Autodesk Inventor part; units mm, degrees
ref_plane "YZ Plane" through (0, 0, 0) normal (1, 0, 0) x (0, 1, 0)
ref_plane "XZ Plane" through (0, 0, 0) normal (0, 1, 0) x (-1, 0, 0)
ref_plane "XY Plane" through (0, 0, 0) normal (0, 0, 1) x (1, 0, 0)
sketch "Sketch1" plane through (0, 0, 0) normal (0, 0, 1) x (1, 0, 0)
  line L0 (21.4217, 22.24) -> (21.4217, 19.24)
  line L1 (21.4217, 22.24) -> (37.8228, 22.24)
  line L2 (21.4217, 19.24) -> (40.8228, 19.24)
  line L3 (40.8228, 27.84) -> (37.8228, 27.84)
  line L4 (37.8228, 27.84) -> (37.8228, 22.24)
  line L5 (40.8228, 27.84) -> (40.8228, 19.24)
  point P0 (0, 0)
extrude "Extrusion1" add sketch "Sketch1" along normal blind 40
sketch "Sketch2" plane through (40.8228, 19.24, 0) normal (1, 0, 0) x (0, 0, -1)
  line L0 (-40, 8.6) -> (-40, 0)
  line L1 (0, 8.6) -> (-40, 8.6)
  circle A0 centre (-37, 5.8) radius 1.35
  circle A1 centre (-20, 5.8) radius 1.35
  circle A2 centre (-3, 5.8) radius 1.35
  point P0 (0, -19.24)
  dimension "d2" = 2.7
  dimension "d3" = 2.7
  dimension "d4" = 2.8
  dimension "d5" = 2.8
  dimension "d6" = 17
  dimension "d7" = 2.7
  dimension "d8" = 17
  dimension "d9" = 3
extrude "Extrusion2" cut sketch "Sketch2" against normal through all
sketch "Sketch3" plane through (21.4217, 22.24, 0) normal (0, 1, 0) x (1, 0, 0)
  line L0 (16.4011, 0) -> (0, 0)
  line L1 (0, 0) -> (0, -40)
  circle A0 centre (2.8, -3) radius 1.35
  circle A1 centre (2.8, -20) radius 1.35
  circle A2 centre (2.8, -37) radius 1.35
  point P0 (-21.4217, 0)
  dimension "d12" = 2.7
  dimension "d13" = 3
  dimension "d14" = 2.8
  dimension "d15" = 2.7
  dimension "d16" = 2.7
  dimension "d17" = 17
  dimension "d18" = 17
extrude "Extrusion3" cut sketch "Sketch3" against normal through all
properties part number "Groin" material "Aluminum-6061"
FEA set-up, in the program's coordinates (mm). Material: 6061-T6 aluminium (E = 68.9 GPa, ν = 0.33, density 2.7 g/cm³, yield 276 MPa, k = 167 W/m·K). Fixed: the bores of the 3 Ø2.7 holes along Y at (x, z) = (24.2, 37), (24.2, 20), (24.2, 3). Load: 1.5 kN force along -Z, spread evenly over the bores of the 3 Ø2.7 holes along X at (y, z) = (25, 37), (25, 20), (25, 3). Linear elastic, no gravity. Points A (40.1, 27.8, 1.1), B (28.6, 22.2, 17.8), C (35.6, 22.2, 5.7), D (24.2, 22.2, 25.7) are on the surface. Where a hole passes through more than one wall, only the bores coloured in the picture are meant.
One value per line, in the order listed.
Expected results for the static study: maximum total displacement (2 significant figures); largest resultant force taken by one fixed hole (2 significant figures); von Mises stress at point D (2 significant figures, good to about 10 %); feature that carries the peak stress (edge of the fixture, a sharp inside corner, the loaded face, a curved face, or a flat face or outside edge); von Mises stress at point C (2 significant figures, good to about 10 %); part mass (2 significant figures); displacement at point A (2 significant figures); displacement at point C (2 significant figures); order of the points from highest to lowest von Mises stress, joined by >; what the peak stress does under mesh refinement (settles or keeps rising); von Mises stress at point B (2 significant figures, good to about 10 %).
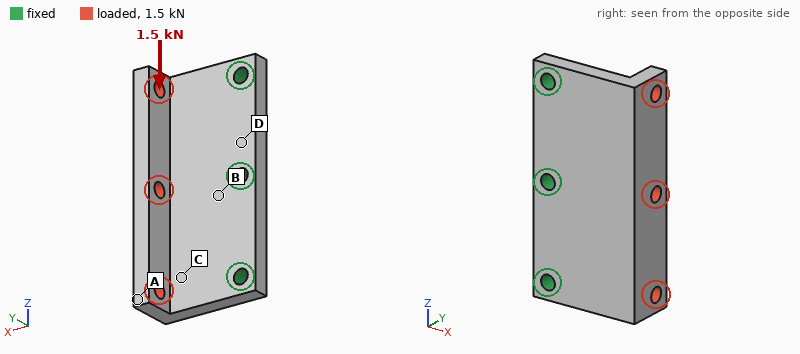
89 µm
790 N
24 MPa
edge of the fixture
65 MPa
7.8 g
84 µm
37 µm
C > B > D > A
keeps rising
51 MPa
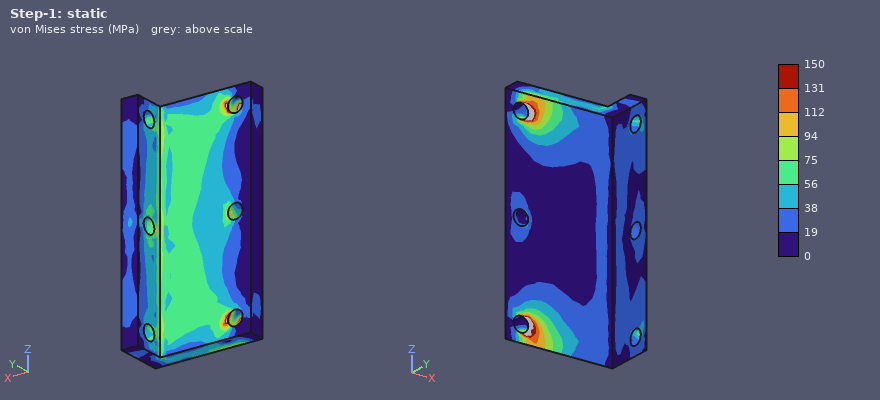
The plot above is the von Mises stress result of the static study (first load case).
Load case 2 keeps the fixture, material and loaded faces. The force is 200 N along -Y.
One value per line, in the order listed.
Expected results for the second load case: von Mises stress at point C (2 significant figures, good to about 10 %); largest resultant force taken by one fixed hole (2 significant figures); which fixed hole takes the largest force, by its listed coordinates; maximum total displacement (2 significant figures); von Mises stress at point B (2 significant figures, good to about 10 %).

13 MPa
86 N
(24.2, 20)
56 µm
35 MPa
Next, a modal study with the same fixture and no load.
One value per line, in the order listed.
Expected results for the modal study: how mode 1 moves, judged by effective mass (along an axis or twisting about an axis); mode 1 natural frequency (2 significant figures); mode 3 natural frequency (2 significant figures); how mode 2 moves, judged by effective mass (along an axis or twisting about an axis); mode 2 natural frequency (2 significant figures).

along Y
5700 Hz
25 kHz
twisting about X
9200 Hz
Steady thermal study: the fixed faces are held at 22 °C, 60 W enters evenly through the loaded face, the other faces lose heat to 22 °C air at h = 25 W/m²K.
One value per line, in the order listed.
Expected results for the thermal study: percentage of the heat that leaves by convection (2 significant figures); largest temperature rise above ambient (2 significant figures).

3.1 %
75 K
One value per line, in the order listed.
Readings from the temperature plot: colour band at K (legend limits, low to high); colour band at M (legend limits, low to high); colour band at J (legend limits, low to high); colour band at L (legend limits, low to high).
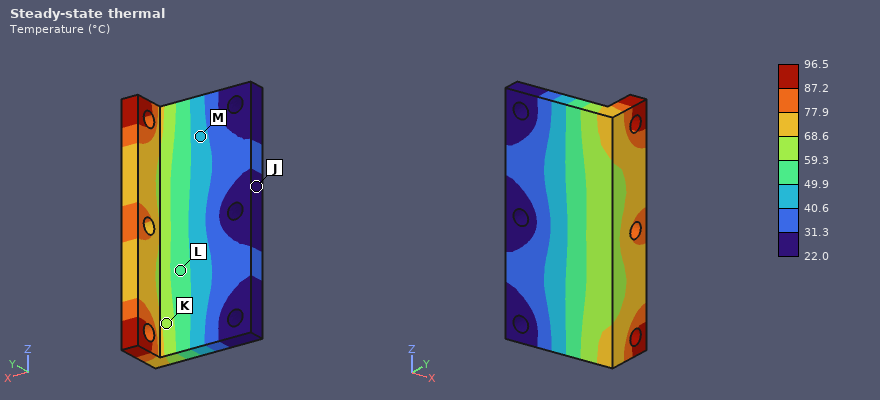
59.3 to 68.6 °C
40.6 to 49.9 °C
22.0 to 31.3 °C
49.9 to 59.3 °C
